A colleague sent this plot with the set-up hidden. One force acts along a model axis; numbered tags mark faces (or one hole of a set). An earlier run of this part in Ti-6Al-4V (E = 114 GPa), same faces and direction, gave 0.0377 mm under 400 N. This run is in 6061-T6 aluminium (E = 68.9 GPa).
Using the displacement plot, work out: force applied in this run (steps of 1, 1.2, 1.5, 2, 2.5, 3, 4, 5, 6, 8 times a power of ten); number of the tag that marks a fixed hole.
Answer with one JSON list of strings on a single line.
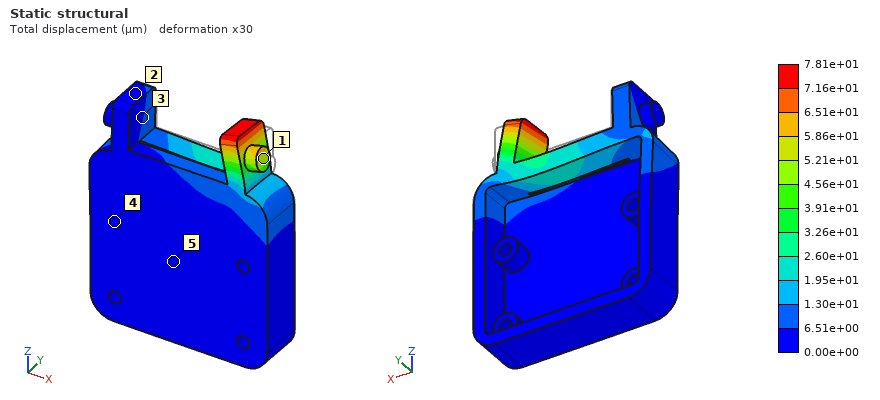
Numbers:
["500 N", "4"]
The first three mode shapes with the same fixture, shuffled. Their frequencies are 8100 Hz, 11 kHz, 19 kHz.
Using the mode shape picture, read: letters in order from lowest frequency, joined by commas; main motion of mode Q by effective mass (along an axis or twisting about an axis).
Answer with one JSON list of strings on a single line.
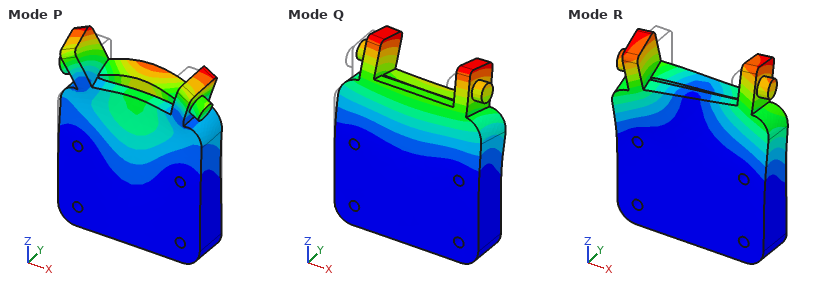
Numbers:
["Q, R, P", "along Y"]
